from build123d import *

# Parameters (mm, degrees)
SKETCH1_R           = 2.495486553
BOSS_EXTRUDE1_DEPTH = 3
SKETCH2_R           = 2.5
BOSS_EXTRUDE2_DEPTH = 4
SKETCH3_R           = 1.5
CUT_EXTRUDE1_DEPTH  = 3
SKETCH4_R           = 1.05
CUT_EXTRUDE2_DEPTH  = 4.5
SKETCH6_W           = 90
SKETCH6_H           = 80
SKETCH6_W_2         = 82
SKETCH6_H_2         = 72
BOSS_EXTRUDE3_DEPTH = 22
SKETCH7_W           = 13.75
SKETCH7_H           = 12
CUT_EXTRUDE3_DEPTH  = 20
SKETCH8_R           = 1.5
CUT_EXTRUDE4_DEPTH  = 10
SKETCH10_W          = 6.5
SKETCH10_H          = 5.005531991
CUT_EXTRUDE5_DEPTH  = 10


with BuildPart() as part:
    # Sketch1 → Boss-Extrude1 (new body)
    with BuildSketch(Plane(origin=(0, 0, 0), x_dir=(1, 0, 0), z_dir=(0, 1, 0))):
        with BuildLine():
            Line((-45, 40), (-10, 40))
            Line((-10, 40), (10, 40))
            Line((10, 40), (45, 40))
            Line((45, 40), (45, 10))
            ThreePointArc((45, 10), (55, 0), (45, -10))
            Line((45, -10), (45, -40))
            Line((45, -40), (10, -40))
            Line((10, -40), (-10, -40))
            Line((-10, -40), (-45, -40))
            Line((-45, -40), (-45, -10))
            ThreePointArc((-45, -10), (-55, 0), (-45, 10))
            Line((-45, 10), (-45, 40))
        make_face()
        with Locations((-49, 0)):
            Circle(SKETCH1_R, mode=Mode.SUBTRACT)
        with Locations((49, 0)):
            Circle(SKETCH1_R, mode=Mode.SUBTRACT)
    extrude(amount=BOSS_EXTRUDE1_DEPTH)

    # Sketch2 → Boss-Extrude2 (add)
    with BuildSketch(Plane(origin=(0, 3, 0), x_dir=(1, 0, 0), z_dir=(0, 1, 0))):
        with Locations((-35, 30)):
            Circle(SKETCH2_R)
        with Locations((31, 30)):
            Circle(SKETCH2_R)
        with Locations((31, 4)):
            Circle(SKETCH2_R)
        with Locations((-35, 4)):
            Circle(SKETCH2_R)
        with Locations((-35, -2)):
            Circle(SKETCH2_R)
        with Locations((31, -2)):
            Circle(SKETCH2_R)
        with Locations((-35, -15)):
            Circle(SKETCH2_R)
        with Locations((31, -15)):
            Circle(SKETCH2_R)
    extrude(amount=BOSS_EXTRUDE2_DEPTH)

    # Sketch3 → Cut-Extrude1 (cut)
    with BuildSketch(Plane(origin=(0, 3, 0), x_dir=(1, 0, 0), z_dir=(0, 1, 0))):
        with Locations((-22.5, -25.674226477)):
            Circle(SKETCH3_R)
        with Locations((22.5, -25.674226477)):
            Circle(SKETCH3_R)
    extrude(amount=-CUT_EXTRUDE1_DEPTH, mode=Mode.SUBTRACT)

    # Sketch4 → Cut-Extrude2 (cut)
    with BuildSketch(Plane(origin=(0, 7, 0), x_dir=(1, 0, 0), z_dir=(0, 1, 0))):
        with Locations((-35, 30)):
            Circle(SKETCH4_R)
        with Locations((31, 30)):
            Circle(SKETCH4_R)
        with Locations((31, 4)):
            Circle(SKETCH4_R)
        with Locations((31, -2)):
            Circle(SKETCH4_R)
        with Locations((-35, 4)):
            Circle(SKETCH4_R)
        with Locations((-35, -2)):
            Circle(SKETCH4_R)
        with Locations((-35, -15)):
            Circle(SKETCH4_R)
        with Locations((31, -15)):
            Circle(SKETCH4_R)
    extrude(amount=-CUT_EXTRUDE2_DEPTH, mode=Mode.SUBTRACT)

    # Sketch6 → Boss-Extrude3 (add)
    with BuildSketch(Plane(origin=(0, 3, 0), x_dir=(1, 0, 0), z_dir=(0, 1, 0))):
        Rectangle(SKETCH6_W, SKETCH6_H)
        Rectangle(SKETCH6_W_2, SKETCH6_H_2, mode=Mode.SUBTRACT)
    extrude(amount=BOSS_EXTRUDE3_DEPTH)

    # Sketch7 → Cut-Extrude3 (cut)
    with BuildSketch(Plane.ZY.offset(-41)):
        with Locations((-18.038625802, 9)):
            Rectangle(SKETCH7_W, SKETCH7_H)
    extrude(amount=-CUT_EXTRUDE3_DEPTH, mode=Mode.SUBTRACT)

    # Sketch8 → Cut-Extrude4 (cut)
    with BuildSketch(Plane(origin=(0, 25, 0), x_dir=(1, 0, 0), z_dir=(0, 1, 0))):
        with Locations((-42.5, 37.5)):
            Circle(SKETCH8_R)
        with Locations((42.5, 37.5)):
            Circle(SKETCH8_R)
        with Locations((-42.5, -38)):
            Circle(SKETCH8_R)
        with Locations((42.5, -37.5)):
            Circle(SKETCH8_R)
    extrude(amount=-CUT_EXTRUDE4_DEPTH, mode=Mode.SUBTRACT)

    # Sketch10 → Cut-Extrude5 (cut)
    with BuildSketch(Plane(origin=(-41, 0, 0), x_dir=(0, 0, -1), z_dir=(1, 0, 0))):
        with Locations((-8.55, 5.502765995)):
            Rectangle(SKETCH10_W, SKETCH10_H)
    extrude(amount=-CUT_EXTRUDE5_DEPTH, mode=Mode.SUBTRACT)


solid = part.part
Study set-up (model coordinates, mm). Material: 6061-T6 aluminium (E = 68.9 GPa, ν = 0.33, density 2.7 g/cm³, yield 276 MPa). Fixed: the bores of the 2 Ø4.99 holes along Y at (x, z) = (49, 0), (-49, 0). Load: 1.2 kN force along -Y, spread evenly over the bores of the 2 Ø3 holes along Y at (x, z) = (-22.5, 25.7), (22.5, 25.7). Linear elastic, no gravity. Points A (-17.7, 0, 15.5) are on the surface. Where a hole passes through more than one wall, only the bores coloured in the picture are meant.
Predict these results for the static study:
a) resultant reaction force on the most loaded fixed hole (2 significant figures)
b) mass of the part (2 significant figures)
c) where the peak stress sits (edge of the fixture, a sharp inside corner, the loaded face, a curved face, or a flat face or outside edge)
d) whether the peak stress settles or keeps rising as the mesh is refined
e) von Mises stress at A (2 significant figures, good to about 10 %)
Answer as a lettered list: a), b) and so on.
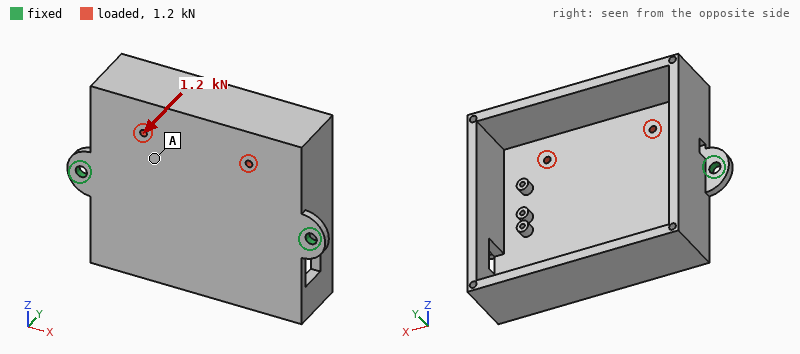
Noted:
a) 610 N
b) 140 g
c) edge of the fixture
d) keeps rising
e) 30 MPa
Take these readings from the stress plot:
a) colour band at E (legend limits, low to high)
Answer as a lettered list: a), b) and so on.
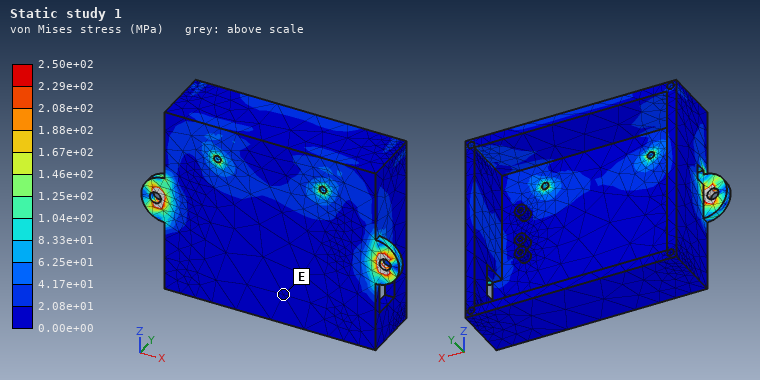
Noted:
a) 0.00e+00 to 2.08e+01 MPa
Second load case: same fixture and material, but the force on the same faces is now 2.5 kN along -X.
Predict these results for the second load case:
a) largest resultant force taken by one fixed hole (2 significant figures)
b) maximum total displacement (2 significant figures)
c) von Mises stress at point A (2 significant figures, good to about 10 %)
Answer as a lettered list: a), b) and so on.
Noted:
a) 1.4 kN
b) 18 µm
c) 16 MPa
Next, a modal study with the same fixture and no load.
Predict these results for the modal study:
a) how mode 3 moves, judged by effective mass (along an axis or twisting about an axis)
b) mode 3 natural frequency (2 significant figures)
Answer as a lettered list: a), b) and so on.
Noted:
a) along Y
b) 2600 Hz
